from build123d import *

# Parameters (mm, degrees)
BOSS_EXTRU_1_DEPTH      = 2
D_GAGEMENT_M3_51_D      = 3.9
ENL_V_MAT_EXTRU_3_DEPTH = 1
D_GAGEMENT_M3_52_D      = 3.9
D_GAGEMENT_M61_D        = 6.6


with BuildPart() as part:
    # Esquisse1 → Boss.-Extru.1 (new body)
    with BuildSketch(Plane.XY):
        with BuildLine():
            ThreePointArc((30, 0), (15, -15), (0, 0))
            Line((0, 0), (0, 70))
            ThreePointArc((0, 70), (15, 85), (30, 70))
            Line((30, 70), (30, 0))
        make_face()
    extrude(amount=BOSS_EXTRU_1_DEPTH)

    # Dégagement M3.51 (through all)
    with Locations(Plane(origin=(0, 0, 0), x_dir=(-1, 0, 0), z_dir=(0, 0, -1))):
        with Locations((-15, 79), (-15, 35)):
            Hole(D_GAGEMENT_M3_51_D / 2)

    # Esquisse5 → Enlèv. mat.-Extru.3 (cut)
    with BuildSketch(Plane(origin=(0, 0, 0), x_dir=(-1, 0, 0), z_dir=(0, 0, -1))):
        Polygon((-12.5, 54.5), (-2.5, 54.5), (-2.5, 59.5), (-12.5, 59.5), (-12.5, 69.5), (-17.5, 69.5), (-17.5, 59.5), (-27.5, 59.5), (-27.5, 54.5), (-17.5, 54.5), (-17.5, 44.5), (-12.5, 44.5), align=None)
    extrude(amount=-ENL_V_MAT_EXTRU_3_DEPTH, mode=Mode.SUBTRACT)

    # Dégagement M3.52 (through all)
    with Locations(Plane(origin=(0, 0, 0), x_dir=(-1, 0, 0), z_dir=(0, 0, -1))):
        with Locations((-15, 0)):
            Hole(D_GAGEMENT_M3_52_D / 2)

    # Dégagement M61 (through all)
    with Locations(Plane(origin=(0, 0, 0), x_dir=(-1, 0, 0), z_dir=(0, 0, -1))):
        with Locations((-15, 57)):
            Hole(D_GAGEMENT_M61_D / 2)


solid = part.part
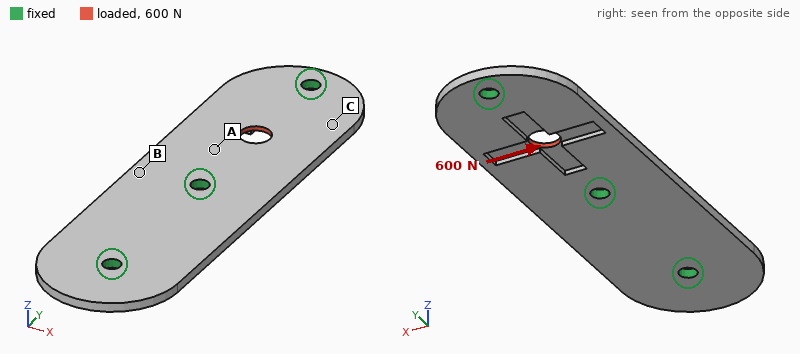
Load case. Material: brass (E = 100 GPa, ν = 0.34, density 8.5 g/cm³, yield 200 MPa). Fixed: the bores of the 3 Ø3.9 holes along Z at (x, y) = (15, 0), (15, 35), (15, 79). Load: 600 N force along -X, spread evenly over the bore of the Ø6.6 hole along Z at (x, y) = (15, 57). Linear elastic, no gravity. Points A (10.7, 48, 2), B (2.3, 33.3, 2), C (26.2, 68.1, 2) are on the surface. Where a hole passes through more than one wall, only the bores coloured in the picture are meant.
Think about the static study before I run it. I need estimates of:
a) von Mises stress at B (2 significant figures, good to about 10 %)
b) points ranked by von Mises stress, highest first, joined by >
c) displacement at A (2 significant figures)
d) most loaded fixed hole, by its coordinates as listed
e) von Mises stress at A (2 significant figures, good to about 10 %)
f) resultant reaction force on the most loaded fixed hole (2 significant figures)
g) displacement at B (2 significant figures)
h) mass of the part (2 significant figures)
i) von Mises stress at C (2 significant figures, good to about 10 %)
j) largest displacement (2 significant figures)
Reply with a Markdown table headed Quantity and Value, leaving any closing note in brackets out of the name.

| Quantity | Value |
|---|---|
| von Mises stress at B | 4.1 MPa |
| points ranked by von Mises stress, highest first, joined by > | A > C > B |
| displacement at A | 5.1 µm |
| most loaded fixed hole, by its coordinates as listed | (15, 35) |
| von Mises stress at A | 18 MPa |
| resultant reaction force on the most loaded fixed hole | 380 N |
| displacement at B | 2.5 µm |
| mass of the part | 45 g |
| von Mises stress at C | 12 MPa |
| largest displacement | 14 µm |
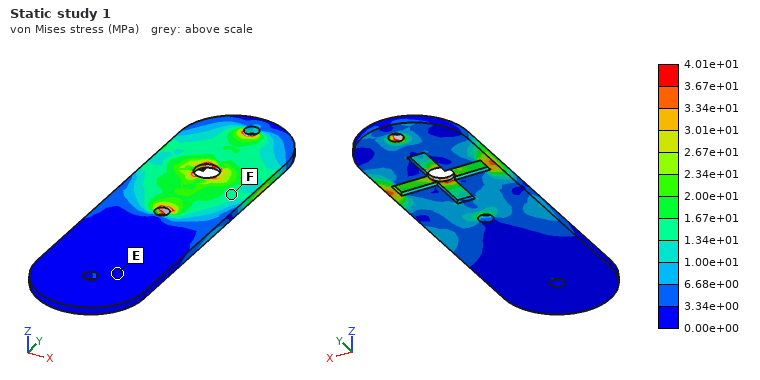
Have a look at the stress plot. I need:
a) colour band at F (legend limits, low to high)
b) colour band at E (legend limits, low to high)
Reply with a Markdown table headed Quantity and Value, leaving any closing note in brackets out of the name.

| Quantity | Value |
|---|---|
| colour band at F | 1.34e+01 to 1.67e+01 MPa |
| colour band at E | 0.00e+00 to 3.34e+00 MPa |
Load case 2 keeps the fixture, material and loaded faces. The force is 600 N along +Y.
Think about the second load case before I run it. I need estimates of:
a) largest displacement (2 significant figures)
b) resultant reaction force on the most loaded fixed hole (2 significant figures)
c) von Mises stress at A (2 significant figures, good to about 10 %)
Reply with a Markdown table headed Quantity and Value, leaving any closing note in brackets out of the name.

| Quantity | Value |
|---|---|
| largest displacement | 3.3 µm |
| resultant reaction force on the most loaded fixed hole | 280 N |
| von Mises stress at A | 14 MPa |
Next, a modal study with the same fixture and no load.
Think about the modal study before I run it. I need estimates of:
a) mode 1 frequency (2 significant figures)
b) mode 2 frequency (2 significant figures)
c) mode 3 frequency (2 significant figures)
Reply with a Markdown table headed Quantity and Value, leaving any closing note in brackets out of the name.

| Quantity | Value |
|---|---|
| mode 1 frequency | 3000 Hz |
| mode 2 frequency | 3000 Hz |
| mode 3 frequency | 3900 Hz |
